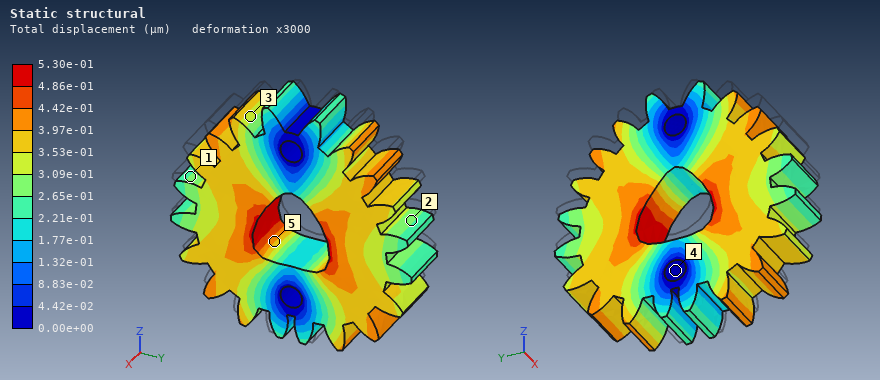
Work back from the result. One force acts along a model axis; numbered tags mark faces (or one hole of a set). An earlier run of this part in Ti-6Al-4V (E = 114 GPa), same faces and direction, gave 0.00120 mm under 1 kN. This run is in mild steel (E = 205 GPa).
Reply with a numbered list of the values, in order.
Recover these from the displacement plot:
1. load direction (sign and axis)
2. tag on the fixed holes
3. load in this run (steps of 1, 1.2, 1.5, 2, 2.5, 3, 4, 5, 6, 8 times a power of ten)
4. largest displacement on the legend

1. -Z
2. 4
3. 800 N
4. 5.30e-01 µm
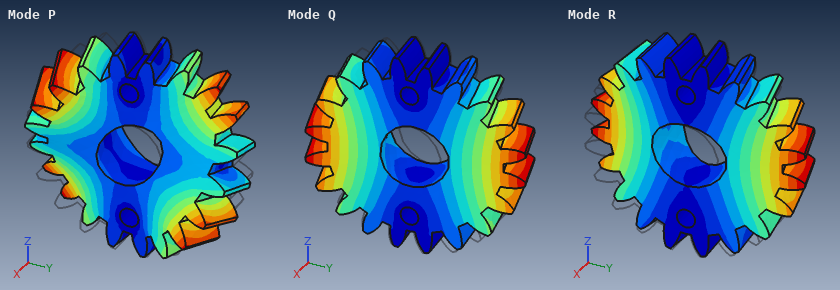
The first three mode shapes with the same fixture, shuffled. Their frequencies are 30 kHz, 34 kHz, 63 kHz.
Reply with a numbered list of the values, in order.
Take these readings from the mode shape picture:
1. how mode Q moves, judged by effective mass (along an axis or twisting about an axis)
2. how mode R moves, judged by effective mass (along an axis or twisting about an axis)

1. twisting about Z
2. along X
